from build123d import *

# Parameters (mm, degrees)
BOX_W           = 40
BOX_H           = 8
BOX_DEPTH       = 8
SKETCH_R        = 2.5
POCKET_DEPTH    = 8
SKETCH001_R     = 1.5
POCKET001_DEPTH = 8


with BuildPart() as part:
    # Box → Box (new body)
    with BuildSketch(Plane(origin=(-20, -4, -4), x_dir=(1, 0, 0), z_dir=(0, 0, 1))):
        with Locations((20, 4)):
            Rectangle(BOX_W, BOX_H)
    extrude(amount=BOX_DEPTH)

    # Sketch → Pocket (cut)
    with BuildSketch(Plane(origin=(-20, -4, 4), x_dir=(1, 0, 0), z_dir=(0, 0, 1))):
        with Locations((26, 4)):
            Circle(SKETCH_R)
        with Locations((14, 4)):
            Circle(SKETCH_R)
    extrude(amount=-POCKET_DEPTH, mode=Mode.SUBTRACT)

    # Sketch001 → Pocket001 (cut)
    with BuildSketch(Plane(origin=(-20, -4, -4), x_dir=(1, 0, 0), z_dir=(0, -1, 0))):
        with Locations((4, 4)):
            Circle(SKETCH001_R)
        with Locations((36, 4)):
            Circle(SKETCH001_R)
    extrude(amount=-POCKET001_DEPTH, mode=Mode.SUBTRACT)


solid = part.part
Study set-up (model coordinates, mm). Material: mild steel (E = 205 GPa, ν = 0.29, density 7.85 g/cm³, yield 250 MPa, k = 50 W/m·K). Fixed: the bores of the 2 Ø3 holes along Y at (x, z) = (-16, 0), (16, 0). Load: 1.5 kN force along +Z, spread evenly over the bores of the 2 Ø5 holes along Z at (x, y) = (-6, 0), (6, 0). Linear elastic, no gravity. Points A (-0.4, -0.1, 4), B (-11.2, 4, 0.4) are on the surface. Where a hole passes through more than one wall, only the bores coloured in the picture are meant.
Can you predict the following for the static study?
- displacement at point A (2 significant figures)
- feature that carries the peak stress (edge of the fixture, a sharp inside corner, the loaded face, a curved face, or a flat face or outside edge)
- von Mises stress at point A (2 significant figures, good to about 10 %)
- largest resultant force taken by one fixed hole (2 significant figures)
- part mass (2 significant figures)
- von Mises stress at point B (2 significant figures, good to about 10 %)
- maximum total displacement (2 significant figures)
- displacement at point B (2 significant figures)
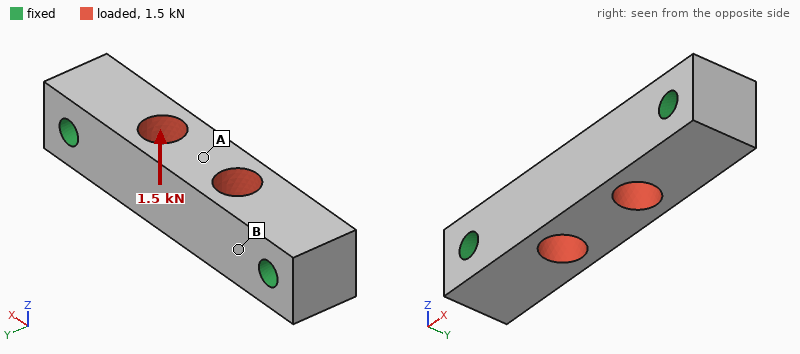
6.4 µm
edge of the fixture
14 MPa
750 N
17 g
36 MPa
6.5 µm
2.0 µm
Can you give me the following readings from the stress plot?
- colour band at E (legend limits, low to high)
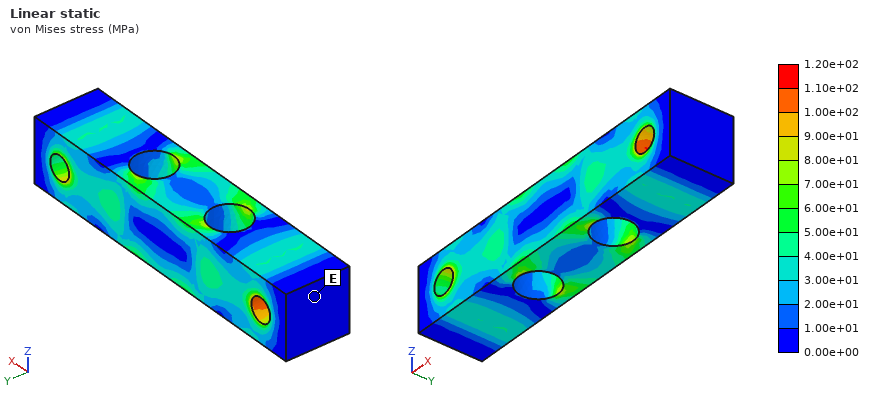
0.00e+00 to 1.00e+01 MPa
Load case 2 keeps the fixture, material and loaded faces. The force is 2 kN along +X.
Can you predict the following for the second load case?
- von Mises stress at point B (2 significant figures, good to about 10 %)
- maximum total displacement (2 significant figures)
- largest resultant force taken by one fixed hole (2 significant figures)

24 MPa
1.4 µm
1.0 kN
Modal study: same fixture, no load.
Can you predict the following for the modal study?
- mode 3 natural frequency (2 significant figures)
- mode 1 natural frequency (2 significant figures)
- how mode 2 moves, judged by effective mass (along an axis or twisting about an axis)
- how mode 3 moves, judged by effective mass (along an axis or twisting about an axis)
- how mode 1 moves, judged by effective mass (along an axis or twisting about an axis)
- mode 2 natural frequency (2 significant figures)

43 kHz
26 kHz
along Z
twisting about X
along Y
28 kHz
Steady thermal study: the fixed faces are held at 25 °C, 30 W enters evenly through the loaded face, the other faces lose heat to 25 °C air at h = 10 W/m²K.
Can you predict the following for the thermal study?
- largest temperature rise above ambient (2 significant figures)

63 K
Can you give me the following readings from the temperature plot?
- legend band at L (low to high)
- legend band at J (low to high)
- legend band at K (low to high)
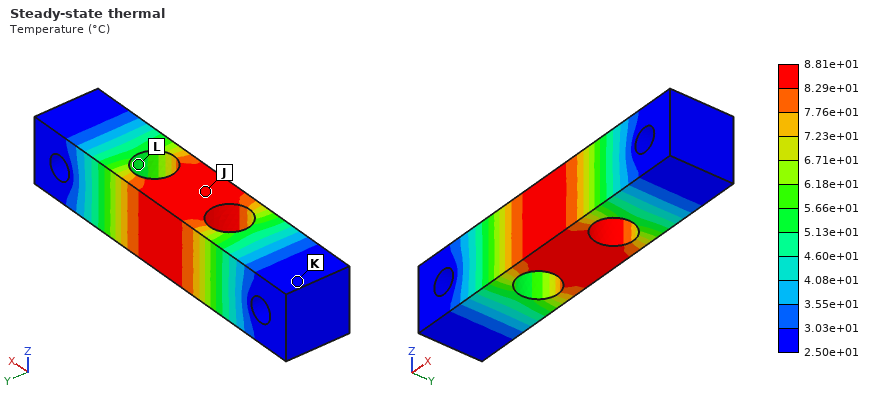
5.13e+01 to 5.66e+01 °C
8.29e+01 to 8.81e+01 °C
2.50e+01 to 3.03e+01 °C
